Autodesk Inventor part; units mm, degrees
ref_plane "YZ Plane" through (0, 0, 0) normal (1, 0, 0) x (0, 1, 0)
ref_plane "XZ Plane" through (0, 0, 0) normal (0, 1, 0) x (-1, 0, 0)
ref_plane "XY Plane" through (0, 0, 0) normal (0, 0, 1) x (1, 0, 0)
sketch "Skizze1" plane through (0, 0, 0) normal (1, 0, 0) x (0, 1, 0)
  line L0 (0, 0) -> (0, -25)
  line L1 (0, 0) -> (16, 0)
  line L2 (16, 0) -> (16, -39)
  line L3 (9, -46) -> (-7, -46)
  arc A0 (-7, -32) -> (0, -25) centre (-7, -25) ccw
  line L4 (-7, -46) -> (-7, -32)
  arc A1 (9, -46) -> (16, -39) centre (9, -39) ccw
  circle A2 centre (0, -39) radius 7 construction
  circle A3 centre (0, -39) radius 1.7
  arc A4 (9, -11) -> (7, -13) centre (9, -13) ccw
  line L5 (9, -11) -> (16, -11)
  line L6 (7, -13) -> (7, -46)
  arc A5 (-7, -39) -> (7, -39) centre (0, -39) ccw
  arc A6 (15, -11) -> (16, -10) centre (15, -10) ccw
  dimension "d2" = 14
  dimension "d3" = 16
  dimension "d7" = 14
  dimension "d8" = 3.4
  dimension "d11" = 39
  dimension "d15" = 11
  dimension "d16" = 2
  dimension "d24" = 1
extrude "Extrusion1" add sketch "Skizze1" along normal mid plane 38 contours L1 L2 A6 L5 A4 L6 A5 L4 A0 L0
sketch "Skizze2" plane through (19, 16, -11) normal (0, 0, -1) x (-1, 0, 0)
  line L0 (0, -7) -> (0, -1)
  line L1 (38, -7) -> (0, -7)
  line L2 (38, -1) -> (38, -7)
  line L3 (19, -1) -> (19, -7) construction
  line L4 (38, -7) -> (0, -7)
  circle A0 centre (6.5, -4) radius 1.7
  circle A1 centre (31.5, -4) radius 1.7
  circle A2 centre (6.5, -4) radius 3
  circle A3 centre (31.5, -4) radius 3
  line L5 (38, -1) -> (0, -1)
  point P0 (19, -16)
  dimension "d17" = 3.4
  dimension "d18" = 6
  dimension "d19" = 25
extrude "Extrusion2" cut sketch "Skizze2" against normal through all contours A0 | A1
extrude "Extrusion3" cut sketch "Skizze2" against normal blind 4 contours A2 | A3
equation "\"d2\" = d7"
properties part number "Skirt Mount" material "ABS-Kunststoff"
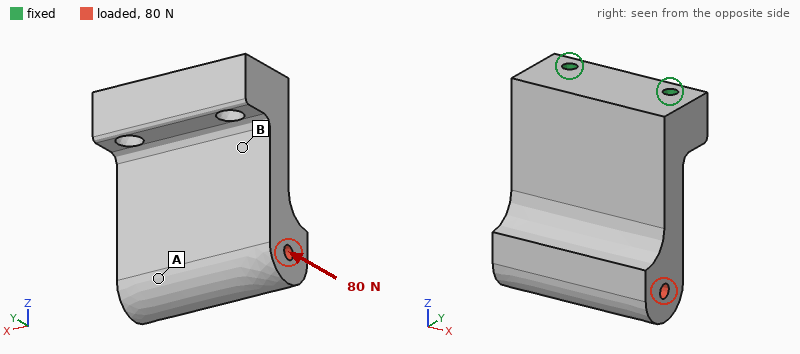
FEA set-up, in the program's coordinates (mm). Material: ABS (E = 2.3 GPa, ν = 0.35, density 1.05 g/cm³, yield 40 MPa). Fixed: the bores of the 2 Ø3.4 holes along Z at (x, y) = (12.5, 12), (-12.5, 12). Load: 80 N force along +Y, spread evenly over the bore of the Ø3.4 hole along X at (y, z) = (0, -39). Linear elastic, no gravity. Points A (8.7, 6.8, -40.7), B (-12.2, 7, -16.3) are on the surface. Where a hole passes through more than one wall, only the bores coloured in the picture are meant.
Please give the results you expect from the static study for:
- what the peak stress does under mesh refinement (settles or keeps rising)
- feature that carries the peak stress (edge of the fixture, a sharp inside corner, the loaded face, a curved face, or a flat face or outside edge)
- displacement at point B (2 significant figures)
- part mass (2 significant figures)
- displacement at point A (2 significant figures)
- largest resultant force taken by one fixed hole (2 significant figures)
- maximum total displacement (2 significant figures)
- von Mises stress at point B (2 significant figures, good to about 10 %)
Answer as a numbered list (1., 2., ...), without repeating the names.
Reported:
1. keeps rising
2. edge of the fixture
3. 0.11 mm
4. 20 g
5. 0.55 mm
6. 48 N
7. 0.67 mm
8. 5.3 MPa
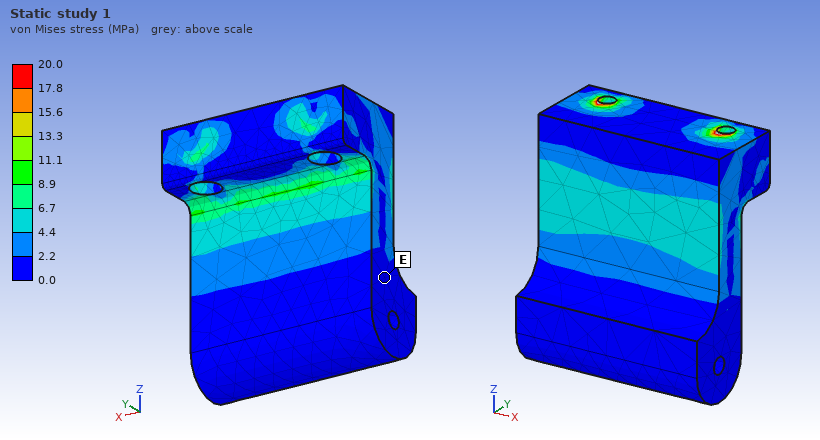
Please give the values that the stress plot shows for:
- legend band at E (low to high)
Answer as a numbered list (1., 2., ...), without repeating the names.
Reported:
1. 0.0 to 2.2 MPa
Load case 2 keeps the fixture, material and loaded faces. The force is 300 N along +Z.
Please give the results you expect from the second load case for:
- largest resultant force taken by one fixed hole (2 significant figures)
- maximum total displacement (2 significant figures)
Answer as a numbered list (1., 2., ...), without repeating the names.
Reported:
1. 150 N
2. 0.58 mm
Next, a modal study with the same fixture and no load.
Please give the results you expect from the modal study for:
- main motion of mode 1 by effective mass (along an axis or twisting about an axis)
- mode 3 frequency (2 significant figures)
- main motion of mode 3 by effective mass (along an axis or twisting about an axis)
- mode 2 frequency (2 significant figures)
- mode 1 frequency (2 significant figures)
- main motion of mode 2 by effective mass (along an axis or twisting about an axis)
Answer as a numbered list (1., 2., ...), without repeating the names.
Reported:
1. along Y
2. 2200 Hz
3. along X
4. 2000 Hz
5. 690 Hz
6. along X
